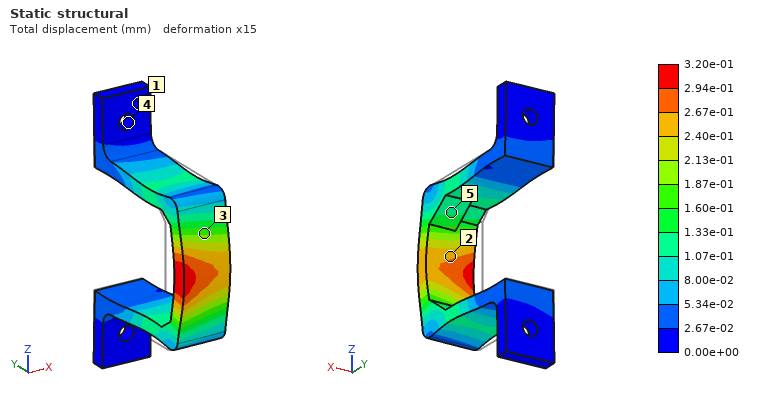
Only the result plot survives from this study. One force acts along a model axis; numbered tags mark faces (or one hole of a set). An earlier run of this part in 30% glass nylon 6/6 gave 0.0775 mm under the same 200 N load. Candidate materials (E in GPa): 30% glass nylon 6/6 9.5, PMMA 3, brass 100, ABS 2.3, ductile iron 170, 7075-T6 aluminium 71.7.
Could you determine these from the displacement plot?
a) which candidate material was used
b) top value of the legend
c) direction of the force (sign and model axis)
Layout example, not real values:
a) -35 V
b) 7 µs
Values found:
a) ABS
b) 3.20e-01 mm
c) -Y
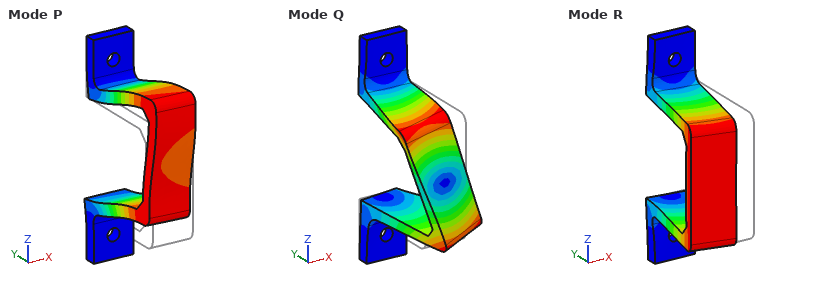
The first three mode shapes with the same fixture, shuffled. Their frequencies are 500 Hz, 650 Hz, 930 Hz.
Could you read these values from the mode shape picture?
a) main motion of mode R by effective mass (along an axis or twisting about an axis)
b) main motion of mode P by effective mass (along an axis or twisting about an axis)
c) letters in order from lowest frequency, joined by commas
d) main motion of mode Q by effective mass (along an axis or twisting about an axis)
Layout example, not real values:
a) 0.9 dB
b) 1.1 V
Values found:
a) along X
b) along Z
c) R, P, Q
d) twisting about Y
